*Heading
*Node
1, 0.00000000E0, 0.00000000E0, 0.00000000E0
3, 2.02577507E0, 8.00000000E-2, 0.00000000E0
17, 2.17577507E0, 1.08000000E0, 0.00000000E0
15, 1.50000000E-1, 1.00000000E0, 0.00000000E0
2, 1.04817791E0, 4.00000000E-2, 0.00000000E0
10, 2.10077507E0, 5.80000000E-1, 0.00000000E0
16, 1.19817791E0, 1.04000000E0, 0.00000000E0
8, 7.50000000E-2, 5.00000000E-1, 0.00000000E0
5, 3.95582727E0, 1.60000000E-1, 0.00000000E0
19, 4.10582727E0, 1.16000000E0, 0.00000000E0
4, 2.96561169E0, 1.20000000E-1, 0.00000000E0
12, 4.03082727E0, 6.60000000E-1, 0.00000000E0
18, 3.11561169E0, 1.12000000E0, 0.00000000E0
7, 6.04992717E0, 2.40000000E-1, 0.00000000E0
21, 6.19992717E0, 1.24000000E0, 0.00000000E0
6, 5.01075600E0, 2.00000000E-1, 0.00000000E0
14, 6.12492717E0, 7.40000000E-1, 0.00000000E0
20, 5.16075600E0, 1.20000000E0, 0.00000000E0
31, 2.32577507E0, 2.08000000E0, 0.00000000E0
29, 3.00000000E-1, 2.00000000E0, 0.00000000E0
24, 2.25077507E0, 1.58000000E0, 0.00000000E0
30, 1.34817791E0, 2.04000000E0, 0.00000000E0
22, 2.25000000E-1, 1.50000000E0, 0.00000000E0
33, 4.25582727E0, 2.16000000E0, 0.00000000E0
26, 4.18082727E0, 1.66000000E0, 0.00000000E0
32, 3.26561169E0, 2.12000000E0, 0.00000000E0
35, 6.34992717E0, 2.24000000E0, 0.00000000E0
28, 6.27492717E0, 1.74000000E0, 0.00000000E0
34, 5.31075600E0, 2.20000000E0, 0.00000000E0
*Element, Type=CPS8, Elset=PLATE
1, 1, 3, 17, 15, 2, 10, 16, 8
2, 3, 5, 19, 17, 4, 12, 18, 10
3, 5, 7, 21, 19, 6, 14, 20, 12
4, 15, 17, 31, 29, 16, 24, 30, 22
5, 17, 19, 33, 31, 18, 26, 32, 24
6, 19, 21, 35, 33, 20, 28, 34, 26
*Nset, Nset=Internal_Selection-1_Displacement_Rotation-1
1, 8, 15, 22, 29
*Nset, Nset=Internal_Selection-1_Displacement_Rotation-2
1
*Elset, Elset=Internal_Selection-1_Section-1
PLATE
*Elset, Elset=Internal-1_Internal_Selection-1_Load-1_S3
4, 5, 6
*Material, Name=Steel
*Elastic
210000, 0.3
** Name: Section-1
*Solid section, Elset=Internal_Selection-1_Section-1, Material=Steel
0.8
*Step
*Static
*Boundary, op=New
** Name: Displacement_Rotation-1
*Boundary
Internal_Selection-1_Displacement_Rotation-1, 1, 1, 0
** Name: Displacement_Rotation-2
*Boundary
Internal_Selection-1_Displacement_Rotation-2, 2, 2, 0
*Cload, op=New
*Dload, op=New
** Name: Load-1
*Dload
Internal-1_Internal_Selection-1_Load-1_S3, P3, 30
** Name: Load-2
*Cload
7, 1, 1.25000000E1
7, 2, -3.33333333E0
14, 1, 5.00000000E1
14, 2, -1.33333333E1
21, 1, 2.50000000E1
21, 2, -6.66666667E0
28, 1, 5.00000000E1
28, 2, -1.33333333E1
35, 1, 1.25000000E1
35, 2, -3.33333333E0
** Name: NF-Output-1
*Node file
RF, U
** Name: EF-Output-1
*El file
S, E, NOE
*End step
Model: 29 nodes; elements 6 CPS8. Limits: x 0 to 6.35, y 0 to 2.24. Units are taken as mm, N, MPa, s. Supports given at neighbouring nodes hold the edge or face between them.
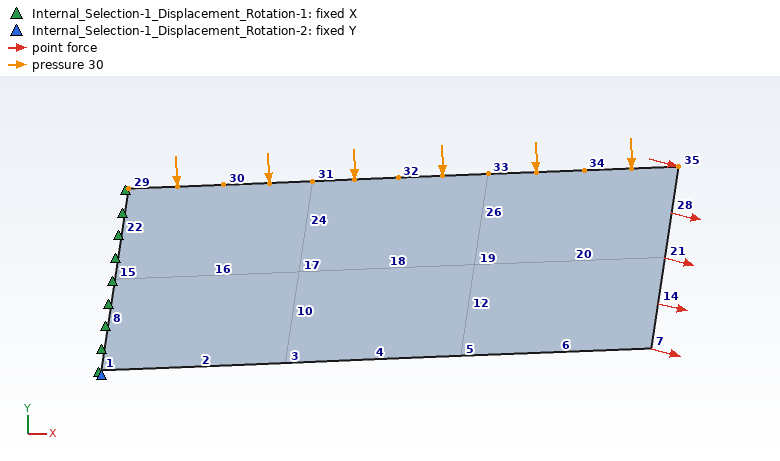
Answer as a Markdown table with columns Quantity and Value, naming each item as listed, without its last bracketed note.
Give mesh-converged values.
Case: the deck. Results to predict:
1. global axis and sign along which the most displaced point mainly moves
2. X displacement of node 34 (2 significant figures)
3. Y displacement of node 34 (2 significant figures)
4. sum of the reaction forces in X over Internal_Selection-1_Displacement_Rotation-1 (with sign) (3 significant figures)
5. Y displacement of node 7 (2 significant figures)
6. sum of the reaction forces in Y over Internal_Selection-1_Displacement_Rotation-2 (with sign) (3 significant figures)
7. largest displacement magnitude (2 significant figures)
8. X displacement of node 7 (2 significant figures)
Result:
| Quantity | Value |
|---|---|
| global axis and sign along which the most displaced point mainly moves | -Y |
| X displacement of node 34 | 0.021 mm |
| Y displacement of node 34 | -0.065 mm |
| sum of the reaction forces in X over Internal_Selection-1_Displacement_Rotation-1 (with sign) | -156 N |
| Y displacement of node 7 | -0.077 mm |
| sum of the reaction forces in Y over Internal_Selection-1_Displacement_Rotation-2 (with sign) | 185 N |
| largest displacement magnitude | 0.086 mm |
| X displacement of node 7 | -0.011 mm |
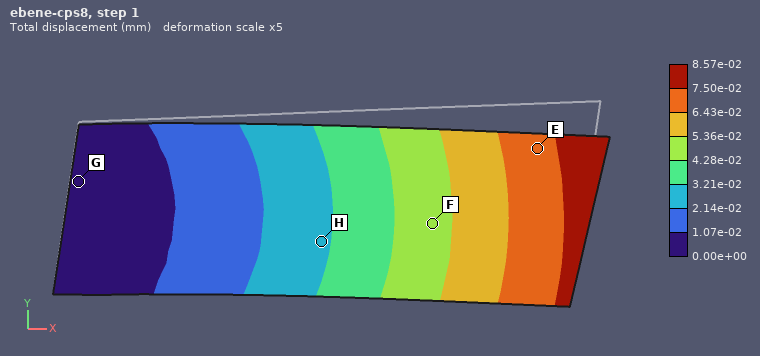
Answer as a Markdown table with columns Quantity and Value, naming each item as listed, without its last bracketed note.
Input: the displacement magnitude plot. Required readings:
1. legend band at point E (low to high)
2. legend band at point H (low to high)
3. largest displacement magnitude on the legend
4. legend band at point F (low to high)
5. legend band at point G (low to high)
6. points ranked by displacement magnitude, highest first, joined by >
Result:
| Quantity | Value |
|---|---|
| legend band at point E | 6.43e-02 to 7.50e-02 mm |
| legend band at point H | 2.14e-02 to 3.21e-02 mm |
| largest displacement magnitude on the legend | 8.57e-02 mm |
| legend band at point F | 4.28e-02 to 5.36e-02 mm |
| legend band at point G | 0.00e+00 to 1.07e-02 mm |
| points ranked by displacement magnitude, highest first, joined by > | E > F > H > G |
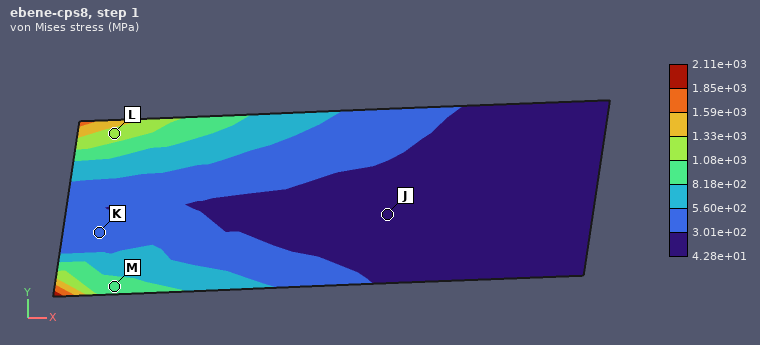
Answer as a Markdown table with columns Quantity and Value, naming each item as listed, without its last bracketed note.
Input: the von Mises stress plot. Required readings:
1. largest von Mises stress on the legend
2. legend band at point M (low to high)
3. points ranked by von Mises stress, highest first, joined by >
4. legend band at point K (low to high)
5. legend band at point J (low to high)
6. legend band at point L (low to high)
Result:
| Quantity | Value |
|---|---|
| largest von Mises stress on the legend | 2.11e+03 MPa |
| legend band at point M | 8.18e+02 to 1.08e+03 MPa |
| points ranked by von Mises stress, highest first, joined by > | L > M > K > J |
| legend band at point K | 3.01e+02 to 5.60e+02 MPa |
| legend band at point J | 4.28e+01 to 3.01e+02 MPa |
| legend band at point L | 1.08e+03 to 1.33e+03 MPa |
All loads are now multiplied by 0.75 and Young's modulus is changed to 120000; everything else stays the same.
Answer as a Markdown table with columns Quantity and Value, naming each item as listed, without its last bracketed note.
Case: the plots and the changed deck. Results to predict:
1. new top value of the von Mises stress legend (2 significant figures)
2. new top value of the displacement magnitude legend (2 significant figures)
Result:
| Quantity | Value |
|---|---|
| new top value of the von Mises stress legend | 1600 MPa |
| new top value of the displacement magnitude legend | 0.11 mm |
